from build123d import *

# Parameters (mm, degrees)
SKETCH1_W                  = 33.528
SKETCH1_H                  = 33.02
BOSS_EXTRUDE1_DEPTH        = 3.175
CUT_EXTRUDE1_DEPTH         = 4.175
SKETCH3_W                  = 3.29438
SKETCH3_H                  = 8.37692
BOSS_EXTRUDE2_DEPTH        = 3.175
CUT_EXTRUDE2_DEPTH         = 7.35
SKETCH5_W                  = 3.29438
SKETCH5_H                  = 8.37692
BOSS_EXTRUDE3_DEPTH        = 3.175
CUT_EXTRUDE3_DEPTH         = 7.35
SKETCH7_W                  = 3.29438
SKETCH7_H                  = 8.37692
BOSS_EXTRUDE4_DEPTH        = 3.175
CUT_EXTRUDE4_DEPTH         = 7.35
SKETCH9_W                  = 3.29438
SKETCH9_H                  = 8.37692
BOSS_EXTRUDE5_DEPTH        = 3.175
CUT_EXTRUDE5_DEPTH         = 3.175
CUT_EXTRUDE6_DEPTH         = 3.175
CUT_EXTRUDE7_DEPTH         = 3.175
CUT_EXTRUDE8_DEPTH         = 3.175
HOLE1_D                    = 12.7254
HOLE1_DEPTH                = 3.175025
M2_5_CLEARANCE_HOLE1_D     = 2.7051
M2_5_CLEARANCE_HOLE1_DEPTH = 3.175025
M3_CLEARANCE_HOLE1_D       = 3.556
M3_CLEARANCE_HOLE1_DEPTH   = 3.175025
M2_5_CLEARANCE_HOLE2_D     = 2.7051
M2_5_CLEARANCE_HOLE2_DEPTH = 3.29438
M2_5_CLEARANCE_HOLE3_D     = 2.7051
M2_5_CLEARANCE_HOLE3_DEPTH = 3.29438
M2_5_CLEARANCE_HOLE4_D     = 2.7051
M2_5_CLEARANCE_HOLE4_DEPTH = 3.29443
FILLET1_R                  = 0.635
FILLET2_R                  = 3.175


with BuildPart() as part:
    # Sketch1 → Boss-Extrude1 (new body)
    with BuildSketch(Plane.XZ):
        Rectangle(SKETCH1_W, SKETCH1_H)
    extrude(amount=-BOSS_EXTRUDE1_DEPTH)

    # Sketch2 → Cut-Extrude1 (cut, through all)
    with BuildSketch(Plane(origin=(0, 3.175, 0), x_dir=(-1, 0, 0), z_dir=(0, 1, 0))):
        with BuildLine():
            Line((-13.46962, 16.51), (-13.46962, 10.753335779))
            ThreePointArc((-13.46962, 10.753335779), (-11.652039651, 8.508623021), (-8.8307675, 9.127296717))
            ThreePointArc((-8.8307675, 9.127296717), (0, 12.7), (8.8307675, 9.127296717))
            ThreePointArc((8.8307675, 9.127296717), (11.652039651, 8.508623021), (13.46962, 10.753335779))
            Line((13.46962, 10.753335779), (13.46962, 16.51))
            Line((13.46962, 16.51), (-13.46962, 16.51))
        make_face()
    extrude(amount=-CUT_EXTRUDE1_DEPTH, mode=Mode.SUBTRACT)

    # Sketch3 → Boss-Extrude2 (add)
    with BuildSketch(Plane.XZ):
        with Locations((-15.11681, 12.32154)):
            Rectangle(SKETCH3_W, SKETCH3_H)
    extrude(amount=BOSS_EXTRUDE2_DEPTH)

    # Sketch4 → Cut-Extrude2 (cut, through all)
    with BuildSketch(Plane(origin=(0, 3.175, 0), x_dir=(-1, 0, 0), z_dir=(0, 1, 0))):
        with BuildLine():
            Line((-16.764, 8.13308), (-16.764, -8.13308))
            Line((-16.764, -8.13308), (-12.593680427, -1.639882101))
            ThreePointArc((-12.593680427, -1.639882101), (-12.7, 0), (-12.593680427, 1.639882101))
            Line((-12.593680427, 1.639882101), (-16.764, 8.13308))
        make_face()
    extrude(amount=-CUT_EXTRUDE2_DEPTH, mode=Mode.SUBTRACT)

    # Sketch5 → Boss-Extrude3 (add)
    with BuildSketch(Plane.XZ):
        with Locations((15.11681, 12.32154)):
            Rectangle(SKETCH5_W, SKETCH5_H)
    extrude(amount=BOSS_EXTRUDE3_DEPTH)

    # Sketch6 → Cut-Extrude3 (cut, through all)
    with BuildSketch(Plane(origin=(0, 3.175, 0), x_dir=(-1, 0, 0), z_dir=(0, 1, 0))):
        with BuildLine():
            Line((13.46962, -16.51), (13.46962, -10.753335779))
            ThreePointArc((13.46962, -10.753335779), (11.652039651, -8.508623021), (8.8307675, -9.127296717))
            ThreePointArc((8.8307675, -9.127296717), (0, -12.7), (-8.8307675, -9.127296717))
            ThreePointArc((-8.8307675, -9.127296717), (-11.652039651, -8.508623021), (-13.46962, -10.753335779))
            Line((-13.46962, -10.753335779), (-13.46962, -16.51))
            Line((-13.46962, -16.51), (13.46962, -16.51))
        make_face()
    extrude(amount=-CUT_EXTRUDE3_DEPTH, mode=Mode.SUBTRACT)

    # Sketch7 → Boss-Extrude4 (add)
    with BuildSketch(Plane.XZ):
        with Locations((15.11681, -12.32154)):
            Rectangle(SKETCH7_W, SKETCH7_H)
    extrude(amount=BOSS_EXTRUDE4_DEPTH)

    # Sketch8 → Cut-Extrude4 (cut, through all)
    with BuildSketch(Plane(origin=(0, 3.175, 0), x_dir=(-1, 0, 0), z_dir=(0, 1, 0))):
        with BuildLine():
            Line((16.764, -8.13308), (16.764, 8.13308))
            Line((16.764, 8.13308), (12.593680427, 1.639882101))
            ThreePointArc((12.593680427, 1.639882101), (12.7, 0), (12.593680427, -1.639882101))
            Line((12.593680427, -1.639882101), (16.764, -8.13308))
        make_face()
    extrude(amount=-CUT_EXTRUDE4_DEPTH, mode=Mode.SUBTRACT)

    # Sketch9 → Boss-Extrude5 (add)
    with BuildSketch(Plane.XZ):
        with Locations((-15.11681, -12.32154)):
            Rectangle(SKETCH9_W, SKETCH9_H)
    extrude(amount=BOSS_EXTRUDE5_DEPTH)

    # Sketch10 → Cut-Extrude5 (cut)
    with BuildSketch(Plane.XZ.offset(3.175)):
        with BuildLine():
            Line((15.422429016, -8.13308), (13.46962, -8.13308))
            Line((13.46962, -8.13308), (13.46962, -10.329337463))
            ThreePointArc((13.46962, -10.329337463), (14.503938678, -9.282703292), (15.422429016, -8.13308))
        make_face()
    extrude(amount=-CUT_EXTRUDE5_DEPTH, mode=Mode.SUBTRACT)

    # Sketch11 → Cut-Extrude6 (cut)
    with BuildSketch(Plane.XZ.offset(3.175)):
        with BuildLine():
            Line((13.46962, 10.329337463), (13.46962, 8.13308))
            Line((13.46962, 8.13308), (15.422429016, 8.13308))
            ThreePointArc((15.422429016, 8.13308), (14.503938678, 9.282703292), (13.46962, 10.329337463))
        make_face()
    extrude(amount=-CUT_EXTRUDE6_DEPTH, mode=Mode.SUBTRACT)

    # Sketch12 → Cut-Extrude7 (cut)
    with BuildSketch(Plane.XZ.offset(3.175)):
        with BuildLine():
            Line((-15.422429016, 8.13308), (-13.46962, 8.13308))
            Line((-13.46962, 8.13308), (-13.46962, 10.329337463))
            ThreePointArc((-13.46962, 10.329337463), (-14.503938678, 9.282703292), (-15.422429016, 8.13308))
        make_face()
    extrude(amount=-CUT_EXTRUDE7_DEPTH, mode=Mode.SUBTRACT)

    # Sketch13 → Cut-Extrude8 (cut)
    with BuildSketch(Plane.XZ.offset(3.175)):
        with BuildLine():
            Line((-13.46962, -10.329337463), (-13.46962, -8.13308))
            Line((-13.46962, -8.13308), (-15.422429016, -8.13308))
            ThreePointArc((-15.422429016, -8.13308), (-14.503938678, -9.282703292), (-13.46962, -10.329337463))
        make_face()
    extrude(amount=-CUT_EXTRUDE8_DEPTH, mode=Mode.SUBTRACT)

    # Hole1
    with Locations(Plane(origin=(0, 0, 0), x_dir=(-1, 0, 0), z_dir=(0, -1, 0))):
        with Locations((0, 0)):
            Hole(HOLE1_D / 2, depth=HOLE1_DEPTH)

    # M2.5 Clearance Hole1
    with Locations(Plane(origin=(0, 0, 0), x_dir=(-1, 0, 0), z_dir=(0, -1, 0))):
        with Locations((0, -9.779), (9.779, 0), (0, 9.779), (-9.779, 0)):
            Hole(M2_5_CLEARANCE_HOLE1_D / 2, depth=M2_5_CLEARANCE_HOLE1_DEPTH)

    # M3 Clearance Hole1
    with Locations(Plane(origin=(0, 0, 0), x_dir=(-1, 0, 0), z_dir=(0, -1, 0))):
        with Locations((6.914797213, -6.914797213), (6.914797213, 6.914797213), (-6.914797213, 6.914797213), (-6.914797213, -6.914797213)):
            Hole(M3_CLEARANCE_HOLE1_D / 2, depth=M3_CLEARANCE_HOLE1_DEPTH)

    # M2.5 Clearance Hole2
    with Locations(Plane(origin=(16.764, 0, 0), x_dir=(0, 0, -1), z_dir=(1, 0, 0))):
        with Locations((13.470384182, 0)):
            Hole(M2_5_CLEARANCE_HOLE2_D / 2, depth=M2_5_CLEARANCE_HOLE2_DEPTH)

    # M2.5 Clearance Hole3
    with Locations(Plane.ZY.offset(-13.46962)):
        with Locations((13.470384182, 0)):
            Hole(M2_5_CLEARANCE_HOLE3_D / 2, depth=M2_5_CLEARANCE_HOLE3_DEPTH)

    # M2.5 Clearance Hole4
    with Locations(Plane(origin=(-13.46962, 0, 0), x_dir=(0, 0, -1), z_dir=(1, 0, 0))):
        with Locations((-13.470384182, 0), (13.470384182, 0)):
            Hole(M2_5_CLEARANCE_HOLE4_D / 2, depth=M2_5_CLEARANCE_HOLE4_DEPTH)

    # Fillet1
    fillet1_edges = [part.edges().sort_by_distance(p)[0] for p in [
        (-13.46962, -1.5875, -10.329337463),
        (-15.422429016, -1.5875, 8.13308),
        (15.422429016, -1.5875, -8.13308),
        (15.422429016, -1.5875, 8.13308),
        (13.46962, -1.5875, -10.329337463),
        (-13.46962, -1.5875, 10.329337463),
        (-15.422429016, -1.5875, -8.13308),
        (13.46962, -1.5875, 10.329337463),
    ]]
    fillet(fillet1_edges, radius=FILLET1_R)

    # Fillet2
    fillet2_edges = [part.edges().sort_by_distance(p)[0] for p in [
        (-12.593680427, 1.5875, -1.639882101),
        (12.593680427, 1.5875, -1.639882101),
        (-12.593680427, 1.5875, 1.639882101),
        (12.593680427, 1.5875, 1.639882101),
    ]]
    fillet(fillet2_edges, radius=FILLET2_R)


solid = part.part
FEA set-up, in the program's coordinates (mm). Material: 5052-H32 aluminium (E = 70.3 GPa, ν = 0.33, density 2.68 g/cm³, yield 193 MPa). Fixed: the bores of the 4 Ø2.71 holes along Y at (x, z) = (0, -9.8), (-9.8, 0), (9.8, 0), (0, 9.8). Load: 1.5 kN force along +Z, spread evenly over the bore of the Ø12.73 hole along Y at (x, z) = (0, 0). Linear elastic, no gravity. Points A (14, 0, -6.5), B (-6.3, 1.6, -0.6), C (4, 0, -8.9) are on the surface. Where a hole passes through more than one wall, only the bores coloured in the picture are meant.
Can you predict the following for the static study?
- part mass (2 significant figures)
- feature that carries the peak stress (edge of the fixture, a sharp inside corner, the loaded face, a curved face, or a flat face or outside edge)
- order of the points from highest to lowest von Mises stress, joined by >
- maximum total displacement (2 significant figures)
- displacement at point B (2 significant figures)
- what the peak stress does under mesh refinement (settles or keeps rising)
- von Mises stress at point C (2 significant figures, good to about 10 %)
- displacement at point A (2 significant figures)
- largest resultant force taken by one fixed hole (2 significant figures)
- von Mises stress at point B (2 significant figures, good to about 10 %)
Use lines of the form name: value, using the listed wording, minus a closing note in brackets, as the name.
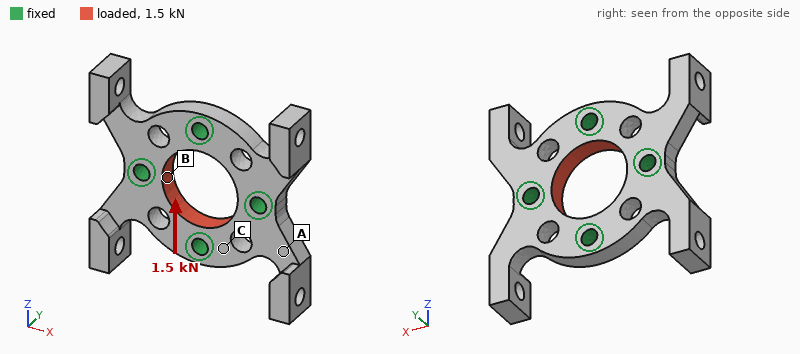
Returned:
part mass: 5.1 g
feature that carries the peak stress: edge of the fixture
order of the points from highest to lowest von Mises stress, joined by >: B > C > A
maximum total displacement: 2.4 µm
displacement at point B: 1.6 µm
what the peak stress does under mesh refinement: keeps rising
von Mises stress at point C: 11 MPa
displacement at point A: 0.80 µm
largest resultant force taken by one fixed hole: 380 N
von Mises stress at point B: 21 MPa
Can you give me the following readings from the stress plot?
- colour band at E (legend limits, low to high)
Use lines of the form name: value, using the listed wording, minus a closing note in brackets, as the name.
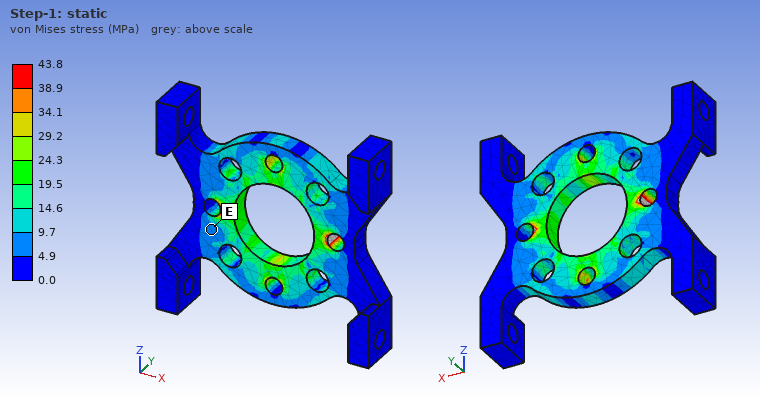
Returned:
colour band at E: 4.9 to 9.7 MPa
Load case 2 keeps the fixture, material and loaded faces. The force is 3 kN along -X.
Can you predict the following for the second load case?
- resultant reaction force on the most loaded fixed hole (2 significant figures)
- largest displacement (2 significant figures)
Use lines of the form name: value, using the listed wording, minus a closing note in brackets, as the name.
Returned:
resultant reaction force on the most loaded fixed hole: 750 N
largest displacement: 4.9 µm
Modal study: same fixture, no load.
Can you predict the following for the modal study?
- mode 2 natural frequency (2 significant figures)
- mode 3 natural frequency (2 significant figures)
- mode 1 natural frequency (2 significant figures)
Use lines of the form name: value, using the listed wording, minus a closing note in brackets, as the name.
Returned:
mode 2 natural frequency: 9300 Hz
mode 3 natural frequency: 9400 Hz
mode 1 natural frequency: 9300 Hz
